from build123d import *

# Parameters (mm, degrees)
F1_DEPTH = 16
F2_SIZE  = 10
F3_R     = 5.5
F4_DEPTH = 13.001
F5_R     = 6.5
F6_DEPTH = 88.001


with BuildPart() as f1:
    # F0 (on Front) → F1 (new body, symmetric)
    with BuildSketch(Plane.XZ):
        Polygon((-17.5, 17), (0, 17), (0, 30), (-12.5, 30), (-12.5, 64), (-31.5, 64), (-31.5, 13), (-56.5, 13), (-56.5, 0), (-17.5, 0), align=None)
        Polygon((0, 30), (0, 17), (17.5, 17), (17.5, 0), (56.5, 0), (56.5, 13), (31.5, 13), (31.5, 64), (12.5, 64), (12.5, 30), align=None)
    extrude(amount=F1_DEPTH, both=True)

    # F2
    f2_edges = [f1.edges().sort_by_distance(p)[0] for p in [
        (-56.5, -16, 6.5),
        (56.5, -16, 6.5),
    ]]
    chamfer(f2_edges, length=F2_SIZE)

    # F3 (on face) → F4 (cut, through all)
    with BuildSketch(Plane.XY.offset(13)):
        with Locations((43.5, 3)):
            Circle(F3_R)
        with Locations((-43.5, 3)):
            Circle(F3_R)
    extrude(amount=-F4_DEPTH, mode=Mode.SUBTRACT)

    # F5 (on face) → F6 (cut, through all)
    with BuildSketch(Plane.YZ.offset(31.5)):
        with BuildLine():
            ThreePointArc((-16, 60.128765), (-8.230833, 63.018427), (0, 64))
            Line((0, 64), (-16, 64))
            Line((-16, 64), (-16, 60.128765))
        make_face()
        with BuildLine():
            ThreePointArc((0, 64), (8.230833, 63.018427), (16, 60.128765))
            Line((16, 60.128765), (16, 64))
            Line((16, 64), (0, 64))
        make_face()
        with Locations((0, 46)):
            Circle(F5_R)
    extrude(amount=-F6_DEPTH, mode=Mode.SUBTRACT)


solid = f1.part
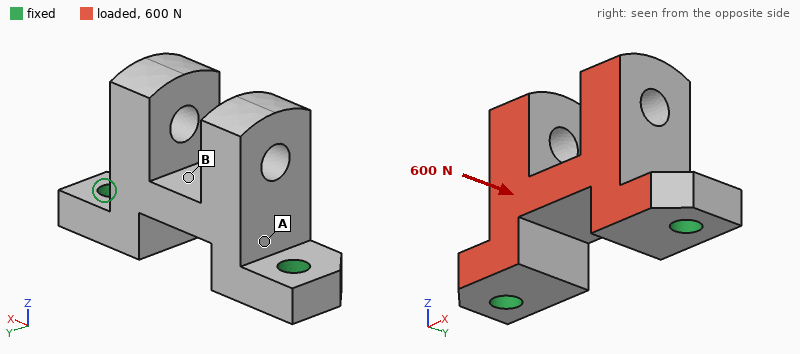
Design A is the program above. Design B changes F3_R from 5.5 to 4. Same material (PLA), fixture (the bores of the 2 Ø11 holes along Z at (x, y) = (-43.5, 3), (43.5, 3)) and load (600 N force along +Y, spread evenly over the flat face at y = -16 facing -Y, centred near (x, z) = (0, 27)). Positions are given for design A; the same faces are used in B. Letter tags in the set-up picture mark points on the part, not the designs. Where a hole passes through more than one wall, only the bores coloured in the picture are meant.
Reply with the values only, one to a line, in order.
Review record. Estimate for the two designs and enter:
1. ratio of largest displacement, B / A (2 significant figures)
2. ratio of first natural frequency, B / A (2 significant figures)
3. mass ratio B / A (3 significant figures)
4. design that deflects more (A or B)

1.2
0.90
1.01
B
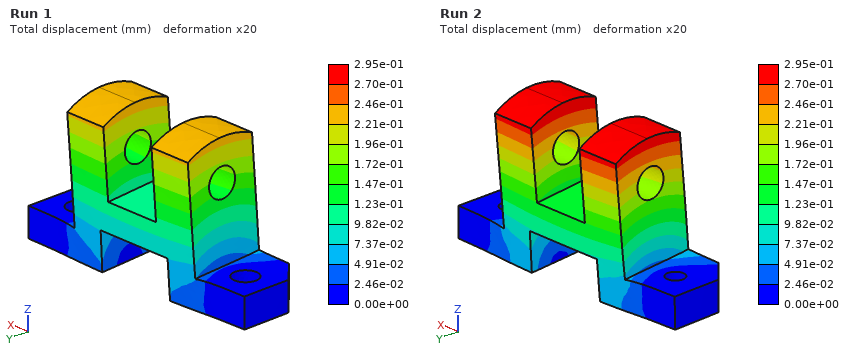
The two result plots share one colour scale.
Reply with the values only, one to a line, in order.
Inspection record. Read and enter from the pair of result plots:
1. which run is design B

Run 2
